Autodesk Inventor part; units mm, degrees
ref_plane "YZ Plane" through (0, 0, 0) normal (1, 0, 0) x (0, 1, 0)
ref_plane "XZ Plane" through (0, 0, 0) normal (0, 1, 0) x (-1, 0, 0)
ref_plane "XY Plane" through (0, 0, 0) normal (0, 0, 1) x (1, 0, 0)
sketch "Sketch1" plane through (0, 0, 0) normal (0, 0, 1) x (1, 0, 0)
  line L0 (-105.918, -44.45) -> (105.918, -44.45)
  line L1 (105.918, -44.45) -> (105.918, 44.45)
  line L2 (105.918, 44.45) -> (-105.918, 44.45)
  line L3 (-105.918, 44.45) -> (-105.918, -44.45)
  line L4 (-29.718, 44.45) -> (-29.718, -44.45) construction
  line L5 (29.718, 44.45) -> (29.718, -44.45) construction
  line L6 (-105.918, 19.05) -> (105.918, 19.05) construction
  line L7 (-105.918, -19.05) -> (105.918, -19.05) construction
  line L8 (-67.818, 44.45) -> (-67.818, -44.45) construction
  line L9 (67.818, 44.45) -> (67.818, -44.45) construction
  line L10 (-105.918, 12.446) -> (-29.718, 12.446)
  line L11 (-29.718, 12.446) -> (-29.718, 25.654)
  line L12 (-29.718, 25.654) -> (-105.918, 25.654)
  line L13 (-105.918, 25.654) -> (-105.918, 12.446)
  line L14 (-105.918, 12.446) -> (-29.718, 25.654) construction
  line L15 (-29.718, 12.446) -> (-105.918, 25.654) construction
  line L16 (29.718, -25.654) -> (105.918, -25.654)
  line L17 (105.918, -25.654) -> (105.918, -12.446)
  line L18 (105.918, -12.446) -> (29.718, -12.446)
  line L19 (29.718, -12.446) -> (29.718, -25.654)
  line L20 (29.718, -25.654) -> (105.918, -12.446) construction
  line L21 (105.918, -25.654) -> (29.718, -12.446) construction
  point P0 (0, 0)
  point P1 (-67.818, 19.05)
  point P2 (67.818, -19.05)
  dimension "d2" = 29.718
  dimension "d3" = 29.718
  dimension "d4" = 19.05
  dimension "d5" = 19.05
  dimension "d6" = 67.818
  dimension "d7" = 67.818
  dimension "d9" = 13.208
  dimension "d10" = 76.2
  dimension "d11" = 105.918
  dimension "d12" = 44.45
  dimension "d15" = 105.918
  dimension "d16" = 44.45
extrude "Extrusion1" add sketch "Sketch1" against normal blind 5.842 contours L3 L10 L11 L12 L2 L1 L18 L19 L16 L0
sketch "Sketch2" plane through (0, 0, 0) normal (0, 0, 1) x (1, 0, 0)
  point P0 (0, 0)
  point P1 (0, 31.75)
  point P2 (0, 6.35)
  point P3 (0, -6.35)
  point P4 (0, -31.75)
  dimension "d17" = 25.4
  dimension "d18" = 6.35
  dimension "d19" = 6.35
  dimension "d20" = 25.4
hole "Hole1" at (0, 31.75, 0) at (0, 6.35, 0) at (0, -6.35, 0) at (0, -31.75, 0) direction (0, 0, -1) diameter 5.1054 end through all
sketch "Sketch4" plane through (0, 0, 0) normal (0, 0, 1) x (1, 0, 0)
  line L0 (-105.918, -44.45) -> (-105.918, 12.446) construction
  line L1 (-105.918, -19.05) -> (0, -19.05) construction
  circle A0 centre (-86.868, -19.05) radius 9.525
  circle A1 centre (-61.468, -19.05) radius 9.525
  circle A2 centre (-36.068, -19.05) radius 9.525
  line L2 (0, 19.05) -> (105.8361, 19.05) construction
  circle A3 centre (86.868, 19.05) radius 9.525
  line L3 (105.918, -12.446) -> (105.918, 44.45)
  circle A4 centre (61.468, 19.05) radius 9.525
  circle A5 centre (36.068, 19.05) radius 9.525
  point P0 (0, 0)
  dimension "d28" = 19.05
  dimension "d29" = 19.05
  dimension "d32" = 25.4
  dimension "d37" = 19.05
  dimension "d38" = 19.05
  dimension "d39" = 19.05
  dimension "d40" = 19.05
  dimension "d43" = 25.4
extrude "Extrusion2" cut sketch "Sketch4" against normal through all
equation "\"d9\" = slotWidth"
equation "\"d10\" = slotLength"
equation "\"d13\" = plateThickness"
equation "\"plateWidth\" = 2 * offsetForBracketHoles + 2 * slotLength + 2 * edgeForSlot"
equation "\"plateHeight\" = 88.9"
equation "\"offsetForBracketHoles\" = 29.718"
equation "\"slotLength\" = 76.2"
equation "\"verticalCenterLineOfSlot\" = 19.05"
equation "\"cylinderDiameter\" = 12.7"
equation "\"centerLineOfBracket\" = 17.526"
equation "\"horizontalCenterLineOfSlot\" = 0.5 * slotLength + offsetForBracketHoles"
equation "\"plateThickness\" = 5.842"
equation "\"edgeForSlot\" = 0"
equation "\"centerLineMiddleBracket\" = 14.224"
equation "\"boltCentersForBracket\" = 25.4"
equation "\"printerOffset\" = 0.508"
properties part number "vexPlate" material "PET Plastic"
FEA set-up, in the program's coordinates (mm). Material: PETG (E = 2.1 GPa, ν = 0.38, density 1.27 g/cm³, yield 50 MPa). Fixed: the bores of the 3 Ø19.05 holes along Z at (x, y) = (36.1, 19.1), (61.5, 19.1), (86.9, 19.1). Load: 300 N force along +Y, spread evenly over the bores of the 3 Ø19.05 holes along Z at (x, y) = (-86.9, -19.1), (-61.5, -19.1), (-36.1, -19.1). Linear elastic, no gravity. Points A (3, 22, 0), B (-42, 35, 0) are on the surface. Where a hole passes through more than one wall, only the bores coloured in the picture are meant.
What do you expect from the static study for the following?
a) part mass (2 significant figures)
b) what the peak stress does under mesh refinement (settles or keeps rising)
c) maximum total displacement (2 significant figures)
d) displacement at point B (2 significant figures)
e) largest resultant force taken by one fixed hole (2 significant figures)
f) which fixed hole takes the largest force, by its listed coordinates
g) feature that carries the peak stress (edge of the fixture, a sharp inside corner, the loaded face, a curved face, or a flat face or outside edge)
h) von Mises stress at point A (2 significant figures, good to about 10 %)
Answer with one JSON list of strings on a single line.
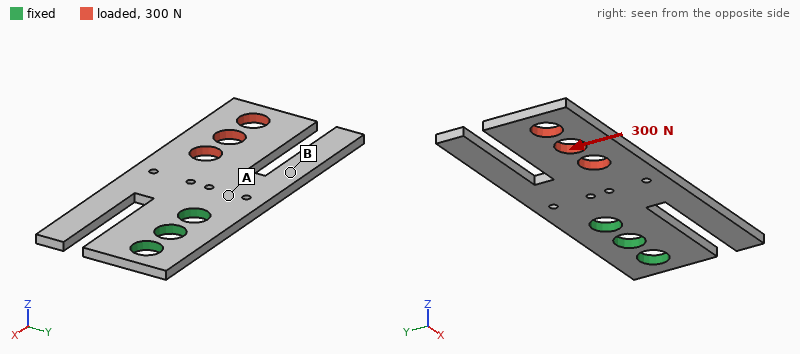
["110 g", "keeps rising", "1.4 mm", "0.48 mm", "660 N", "(36.1, 19.1)", "a sharp inside corner", "4.0 MPa"]
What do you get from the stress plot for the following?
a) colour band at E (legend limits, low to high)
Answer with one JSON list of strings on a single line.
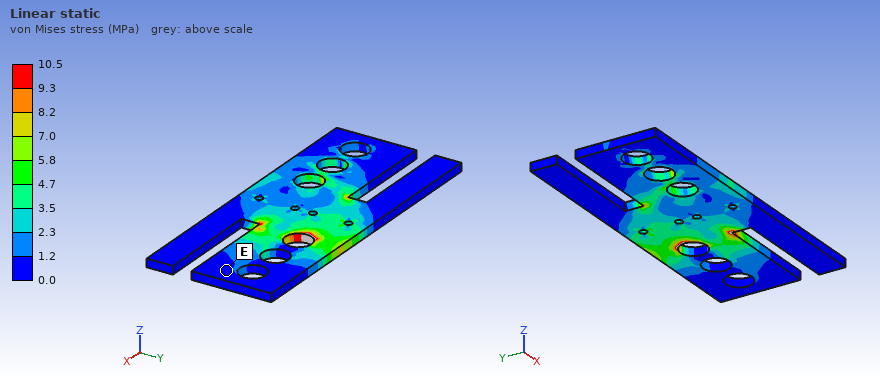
["0.0 to 1.2 MPa"]
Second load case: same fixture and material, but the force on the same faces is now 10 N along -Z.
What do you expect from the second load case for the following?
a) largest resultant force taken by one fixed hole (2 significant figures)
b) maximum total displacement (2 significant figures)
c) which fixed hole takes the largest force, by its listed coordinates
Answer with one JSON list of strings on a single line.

["15 N", "2.6 mm", "(36.1, 19.1)"]
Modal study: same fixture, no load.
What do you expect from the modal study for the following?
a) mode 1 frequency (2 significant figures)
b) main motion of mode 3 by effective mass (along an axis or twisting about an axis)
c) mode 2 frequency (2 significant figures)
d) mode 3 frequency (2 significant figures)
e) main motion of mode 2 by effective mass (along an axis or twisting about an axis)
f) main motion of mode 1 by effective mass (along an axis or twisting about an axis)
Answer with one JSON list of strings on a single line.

["65 Hz", "along Z", "120 Hz", "130 Hz", "twisting about X", "along Z"]
